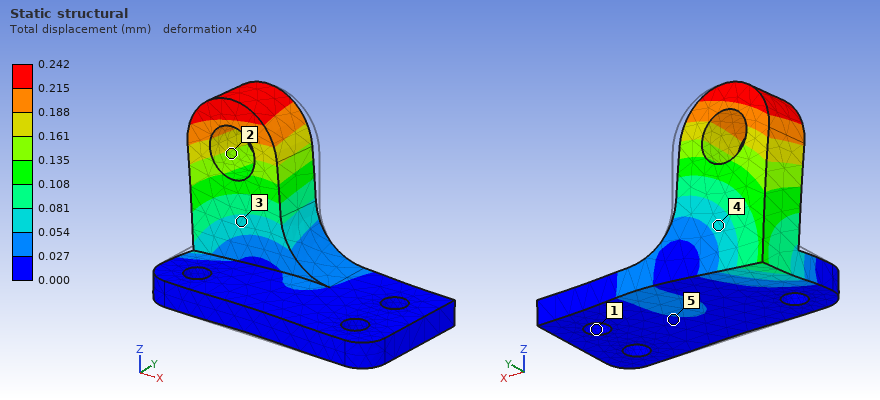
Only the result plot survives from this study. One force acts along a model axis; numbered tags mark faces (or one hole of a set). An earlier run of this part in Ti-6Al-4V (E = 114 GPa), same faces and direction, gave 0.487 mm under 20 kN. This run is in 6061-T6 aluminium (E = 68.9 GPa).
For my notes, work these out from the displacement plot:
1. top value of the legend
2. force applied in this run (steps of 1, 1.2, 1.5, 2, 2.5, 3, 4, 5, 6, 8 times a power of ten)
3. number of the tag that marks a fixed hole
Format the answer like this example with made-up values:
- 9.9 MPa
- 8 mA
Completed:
- 0.242 mm
- 6 kN
- 1
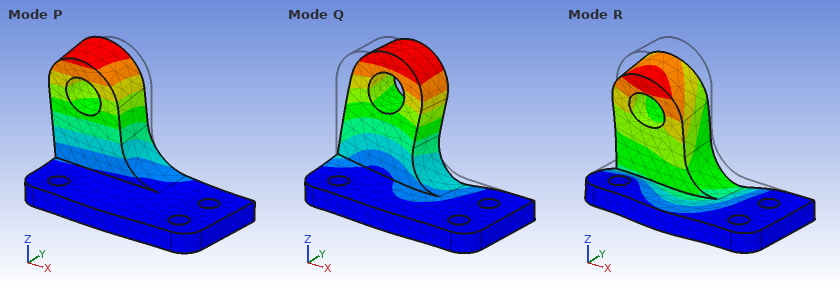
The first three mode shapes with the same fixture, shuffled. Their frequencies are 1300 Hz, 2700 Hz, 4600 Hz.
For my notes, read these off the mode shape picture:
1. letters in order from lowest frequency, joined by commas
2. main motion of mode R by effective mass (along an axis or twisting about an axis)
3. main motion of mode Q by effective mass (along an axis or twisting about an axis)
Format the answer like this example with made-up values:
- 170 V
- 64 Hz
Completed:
- P, Q, R
- along Z
- along X
